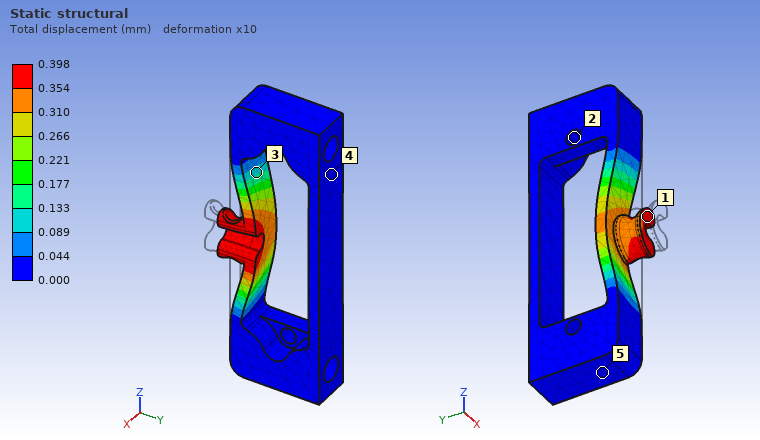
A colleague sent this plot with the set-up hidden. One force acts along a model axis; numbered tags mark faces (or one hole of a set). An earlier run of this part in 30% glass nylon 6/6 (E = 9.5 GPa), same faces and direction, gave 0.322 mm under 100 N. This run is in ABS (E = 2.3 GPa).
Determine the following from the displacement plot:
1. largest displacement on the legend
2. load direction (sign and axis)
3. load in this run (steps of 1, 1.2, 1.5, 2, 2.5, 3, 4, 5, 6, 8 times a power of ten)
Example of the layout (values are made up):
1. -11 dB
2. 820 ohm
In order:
1. 0.398 mm
2. +Y
3. 30 N
